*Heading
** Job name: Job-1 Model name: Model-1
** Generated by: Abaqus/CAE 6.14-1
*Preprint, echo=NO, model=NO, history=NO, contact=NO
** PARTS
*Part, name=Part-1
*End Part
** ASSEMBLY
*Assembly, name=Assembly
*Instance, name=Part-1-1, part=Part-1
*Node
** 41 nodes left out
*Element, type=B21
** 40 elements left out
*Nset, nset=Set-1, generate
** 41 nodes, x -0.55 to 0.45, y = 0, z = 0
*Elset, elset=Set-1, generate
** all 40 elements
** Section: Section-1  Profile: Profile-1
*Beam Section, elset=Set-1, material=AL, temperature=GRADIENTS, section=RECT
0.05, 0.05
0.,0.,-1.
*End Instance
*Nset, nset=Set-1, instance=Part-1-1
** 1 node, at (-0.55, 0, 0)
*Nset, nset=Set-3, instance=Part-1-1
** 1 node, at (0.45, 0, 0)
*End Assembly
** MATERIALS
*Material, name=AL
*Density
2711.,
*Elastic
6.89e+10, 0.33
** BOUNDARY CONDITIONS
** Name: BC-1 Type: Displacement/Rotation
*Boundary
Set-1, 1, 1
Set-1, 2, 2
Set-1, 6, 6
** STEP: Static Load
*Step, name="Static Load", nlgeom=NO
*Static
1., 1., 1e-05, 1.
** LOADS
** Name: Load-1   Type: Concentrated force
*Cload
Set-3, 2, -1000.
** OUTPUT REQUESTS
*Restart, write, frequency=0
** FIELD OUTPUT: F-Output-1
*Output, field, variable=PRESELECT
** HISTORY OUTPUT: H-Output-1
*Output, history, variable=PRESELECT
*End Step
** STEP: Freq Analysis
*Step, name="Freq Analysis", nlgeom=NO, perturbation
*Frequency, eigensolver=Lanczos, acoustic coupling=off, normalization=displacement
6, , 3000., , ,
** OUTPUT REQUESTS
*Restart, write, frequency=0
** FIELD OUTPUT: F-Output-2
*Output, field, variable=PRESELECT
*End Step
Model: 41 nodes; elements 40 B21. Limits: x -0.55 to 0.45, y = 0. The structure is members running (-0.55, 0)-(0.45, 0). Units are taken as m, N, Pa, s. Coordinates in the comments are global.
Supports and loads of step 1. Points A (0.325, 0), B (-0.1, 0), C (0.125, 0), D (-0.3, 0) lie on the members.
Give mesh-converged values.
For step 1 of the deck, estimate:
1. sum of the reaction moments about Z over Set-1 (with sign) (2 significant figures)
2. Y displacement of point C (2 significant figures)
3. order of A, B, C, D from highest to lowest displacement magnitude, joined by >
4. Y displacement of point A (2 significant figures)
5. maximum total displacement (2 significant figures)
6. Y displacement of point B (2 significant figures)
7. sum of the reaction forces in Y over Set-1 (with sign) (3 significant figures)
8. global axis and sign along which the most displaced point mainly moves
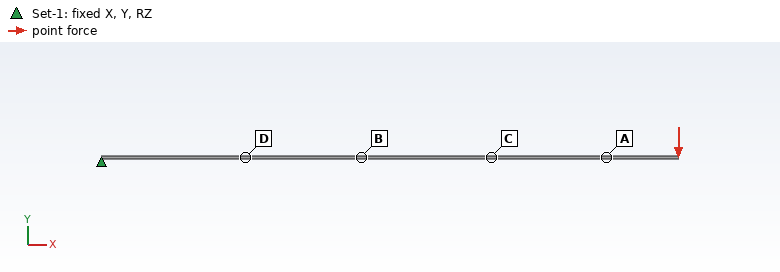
1000 N·m
-0.0049 m
A > C > B > D
-0.0076 m
0.0093 m
-0.0024 m
1000 N
-Y
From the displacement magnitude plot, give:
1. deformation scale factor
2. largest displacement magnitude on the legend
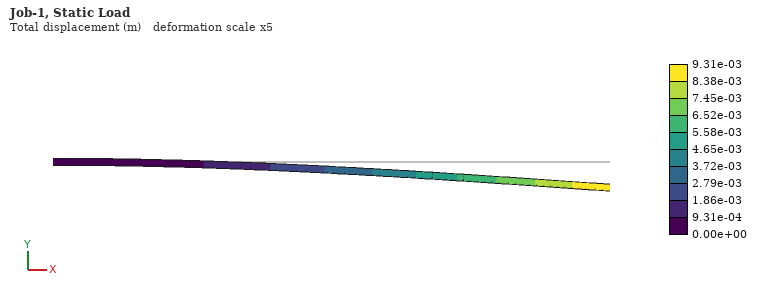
5
9.31e-03 m
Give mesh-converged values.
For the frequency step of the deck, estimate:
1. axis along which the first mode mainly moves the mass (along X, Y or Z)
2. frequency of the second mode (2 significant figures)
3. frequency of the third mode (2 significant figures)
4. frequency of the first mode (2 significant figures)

along Y
250 Hz
690 Hz
41 Hz
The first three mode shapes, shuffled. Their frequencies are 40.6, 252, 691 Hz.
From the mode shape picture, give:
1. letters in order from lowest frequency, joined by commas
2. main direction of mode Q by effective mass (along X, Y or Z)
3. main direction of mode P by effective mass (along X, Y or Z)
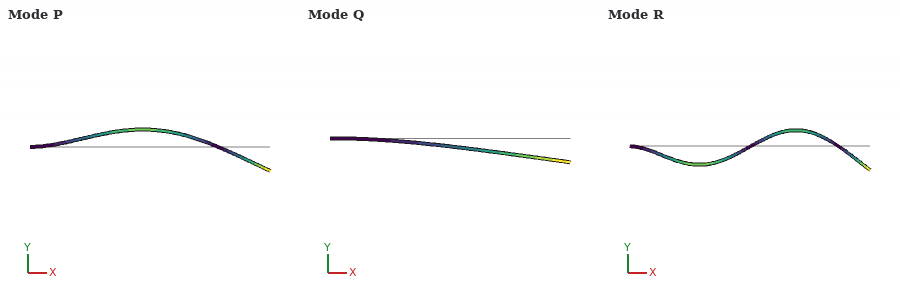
Q, P, R
along Y
along Y
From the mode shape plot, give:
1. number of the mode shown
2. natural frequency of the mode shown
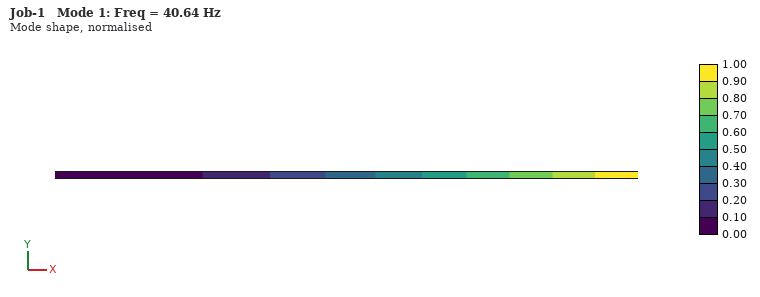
1
40.64 Hz
